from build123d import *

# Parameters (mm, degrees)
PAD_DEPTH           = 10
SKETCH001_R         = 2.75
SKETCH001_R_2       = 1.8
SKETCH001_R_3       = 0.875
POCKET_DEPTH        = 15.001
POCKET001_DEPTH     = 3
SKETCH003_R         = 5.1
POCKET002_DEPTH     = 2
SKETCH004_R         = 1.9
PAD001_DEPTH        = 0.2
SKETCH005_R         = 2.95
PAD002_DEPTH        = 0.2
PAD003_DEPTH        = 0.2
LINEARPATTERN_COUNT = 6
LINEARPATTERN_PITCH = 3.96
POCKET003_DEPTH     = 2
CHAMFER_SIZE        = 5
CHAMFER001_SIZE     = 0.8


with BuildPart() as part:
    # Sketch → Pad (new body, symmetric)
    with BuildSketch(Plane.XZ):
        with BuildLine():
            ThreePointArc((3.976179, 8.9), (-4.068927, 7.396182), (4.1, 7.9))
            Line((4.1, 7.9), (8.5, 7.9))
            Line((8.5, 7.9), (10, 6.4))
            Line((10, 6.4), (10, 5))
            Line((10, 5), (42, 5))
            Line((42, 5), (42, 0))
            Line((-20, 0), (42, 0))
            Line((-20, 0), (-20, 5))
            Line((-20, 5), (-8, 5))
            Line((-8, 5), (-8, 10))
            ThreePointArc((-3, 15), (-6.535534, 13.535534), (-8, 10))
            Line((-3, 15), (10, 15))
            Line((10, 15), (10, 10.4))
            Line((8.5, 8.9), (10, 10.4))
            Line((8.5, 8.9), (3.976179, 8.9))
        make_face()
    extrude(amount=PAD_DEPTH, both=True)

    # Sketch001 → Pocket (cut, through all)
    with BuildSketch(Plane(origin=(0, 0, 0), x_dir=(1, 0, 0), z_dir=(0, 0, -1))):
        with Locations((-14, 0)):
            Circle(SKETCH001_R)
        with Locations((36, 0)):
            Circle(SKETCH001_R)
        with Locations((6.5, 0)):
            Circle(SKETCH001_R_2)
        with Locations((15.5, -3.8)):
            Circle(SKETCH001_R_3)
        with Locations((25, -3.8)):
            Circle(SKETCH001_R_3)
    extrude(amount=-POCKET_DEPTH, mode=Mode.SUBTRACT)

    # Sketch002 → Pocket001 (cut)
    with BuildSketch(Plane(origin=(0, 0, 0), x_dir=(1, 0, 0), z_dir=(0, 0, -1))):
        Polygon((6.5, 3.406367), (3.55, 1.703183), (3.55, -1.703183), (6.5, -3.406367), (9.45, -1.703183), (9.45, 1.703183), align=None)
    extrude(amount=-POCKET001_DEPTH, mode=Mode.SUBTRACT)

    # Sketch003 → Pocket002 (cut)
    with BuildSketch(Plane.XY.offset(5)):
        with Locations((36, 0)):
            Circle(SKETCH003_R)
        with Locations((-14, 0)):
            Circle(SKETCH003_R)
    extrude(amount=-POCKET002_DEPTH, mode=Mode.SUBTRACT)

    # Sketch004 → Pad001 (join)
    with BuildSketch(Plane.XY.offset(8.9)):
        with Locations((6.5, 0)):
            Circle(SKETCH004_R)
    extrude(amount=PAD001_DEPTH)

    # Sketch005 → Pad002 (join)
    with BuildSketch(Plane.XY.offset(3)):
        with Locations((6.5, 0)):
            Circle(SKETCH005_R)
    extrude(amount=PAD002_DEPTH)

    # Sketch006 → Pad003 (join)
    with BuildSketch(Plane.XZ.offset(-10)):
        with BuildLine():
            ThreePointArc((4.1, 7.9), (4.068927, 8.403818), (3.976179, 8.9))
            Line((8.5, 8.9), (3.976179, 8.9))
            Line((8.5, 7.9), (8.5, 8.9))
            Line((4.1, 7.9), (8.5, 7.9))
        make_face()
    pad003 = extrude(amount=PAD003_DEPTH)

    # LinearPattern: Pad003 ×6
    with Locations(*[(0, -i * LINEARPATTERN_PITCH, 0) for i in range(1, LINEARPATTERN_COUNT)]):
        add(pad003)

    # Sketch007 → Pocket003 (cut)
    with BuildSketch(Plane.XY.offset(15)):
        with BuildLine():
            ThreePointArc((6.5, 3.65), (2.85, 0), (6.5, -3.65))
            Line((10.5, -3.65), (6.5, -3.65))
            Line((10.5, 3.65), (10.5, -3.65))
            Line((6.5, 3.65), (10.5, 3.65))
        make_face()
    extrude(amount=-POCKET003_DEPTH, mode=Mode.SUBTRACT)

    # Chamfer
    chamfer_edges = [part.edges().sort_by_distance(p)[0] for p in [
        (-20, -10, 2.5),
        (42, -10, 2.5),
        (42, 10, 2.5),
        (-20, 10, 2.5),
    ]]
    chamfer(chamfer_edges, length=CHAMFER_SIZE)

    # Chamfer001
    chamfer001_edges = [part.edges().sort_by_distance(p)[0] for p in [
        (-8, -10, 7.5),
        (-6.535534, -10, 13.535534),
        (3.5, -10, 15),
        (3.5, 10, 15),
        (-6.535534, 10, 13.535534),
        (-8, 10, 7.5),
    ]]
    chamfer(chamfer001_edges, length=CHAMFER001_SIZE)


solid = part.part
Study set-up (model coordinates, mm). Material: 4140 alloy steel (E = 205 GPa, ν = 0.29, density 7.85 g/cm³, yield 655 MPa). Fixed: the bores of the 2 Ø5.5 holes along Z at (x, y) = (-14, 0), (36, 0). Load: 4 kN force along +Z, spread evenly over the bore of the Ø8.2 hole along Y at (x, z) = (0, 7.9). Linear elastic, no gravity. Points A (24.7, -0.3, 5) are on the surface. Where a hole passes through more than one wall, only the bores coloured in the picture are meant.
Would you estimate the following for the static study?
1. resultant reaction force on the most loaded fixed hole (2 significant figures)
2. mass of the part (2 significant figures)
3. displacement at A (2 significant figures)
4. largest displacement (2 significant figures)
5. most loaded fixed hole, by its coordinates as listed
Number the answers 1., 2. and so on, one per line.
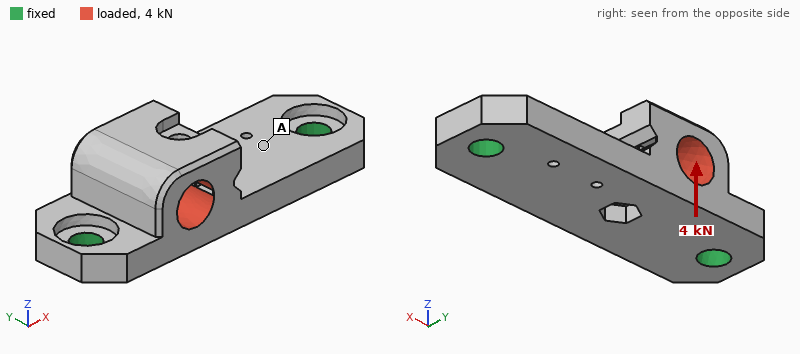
1. 3.5 kN
2. 58 g
3. 20 µm
4. 60 µm
5. (-14, 0)
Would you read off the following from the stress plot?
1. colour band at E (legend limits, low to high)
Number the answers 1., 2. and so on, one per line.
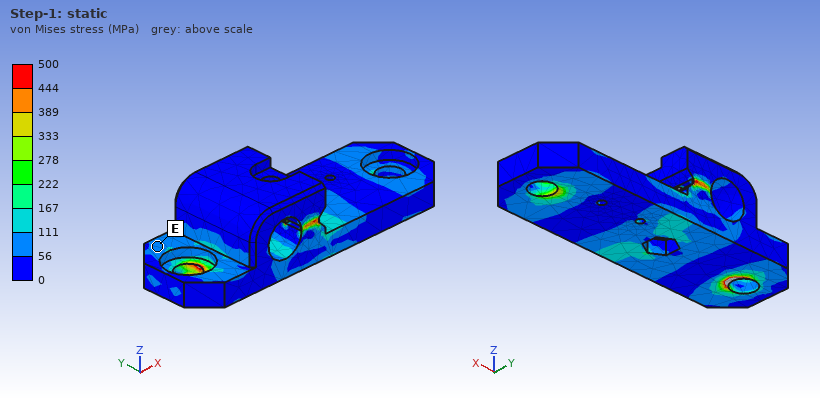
1. 56 to 111 MPa
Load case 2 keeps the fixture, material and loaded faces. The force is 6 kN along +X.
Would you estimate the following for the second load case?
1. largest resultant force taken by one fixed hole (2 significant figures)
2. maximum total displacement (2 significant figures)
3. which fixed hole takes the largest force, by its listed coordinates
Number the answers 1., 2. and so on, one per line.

1. 3.3 kN
2. 45 µm
3. (-14, 0)
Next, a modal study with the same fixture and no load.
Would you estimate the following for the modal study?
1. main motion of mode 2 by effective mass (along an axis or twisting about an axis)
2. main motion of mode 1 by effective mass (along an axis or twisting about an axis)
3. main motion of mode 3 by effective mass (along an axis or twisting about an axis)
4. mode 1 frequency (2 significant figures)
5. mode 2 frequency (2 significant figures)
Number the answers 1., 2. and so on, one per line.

1. along Y
2. along Z
3. along Y
4. 7000 Hz
5. 7600 Hz
